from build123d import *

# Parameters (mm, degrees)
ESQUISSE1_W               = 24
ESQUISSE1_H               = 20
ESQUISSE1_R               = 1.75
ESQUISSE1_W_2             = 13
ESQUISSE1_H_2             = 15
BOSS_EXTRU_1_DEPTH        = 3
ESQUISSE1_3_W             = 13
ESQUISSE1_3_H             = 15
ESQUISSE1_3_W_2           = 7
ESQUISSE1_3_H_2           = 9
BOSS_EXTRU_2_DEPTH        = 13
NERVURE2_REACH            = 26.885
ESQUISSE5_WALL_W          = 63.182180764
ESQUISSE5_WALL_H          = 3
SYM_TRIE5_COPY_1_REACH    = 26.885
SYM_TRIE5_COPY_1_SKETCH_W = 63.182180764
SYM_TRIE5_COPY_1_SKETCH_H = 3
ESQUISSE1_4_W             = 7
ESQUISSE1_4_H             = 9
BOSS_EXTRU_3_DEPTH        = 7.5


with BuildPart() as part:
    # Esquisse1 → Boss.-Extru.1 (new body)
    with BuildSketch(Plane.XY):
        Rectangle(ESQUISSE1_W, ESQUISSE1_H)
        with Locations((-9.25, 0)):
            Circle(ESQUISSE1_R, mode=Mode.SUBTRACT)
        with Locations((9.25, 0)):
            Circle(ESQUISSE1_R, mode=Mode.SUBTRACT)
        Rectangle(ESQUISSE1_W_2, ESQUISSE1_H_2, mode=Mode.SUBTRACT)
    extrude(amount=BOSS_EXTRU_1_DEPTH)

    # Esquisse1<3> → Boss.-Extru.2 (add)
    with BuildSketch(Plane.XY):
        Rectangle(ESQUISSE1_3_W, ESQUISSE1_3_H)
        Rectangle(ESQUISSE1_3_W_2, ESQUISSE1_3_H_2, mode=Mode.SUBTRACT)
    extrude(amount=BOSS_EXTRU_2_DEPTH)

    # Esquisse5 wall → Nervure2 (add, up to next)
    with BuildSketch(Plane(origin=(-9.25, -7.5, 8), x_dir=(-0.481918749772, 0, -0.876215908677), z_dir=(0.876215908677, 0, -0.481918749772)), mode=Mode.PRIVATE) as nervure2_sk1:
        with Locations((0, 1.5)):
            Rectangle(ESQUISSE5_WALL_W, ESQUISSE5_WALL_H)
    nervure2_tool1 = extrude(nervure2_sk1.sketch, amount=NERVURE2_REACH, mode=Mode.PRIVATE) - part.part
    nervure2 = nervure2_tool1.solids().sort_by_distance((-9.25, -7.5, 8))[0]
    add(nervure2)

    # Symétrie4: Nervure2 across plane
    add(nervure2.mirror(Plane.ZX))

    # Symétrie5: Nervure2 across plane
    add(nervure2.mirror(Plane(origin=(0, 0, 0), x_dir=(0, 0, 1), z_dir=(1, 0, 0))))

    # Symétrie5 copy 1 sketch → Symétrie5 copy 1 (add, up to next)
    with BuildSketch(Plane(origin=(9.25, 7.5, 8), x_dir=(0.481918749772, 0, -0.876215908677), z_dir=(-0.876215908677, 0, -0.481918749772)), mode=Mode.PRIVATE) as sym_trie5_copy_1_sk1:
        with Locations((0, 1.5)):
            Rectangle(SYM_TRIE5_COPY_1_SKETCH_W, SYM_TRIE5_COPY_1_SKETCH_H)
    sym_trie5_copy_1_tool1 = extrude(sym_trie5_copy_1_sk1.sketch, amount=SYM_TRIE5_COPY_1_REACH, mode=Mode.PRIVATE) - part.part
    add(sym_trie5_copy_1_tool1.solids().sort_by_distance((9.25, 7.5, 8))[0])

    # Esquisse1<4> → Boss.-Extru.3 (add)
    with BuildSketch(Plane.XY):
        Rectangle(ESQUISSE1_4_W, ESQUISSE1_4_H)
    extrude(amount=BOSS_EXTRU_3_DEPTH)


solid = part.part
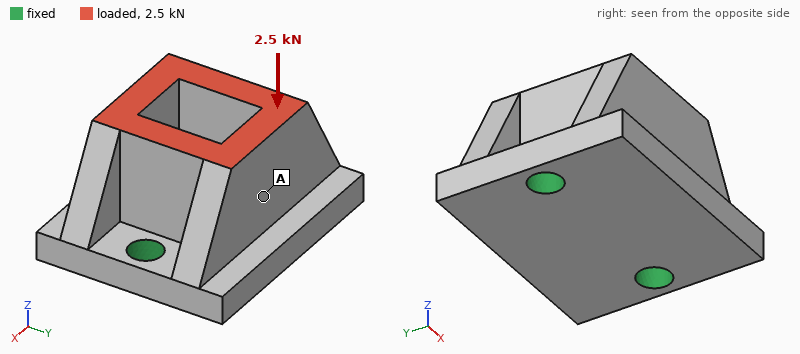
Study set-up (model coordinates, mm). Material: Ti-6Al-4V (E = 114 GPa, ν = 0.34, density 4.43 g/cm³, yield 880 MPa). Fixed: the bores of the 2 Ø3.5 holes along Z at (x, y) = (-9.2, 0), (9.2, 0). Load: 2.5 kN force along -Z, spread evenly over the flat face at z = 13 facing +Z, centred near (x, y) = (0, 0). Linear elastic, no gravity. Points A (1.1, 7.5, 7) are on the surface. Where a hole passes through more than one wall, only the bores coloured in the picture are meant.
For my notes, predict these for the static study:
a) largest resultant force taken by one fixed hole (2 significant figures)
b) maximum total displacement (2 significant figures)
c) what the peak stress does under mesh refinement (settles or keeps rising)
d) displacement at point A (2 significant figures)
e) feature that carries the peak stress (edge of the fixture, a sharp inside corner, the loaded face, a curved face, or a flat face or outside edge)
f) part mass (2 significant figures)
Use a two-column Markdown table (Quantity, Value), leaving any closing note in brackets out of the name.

| Quantity | Value |
|---|---|
| largest resultant force taken by one fixed hole | 1.3 kN |
| maximum total displacement | 6.2 µm |
| what the peak stress does under mesh refinement | keeps rising |
| displacement at point A | 5.6 µm |
| feature that carries the peak stress | edge of the fixture |
| part mass | 15 g |
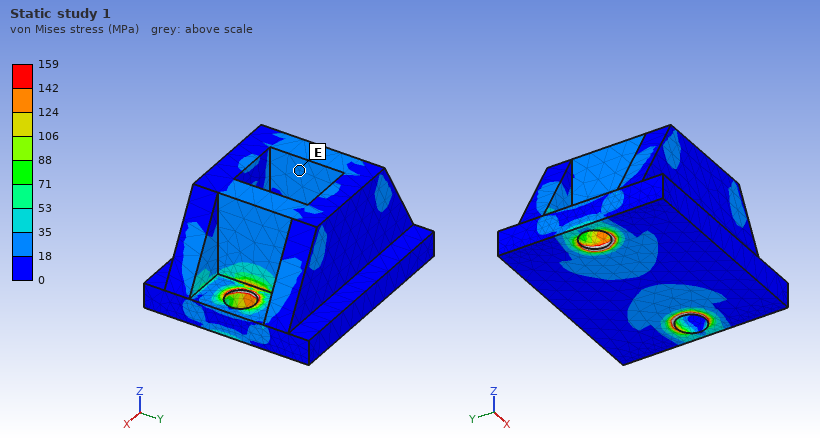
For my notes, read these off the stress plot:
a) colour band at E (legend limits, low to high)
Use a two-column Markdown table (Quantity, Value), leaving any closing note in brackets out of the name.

| Quantity | Value |
|---|---|
| colour band at E | 18 to 35 MPa |
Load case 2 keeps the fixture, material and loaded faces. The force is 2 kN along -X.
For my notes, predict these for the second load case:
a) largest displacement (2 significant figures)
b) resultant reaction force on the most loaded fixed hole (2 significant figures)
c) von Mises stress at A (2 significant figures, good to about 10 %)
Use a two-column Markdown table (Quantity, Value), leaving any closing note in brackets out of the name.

| Quantity | Value |
|---|---|
| largest displacement | 17 µm |
| resultant reaction force on the most loaded fixed hole | 1.7 kN |
| von Mises stress at A | 27 MPa |
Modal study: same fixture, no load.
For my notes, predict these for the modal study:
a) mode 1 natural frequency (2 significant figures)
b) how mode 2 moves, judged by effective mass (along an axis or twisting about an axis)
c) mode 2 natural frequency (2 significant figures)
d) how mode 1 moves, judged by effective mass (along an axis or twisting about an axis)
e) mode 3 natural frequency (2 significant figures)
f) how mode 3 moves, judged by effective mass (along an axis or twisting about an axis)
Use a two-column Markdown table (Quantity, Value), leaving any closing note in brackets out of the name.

| Quantity | Value |
|---|---|
| mode 1 natural frequency | 13 kHz |
| how mode 2 moves, judged by effective mass | along Z |
| mode 2 natural frequency | 31 kHz |
| how mode 1 moves, judged by effective mass | along Y |
| mode 3 natural frequency | 32 kHz |
| how mode 3 moves, judged by effective mass | along X |
